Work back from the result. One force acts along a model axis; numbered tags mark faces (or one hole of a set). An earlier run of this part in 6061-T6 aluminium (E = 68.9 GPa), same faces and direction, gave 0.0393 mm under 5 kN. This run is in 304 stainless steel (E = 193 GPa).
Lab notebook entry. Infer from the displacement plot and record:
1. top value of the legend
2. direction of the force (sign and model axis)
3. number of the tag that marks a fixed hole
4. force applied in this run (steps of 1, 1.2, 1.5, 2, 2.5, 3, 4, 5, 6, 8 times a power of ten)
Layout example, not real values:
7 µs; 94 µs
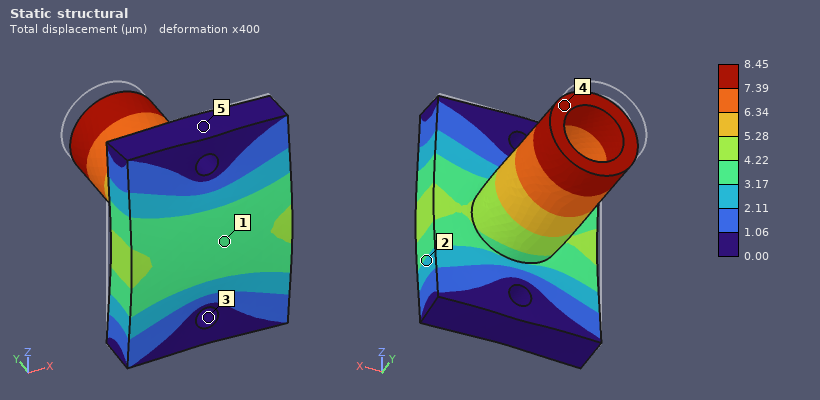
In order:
8.45 µm; -Y; 3; 3 kN
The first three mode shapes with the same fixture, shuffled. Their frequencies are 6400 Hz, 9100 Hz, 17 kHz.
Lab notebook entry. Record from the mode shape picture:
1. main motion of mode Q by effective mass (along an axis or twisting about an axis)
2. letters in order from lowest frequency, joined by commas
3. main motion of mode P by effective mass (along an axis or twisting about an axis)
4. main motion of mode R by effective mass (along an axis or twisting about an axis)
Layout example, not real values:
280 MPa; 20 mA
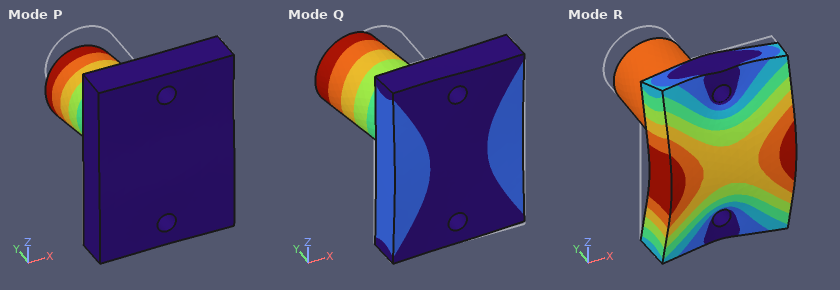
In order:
along X; Q, P, R; along Z; along Y
